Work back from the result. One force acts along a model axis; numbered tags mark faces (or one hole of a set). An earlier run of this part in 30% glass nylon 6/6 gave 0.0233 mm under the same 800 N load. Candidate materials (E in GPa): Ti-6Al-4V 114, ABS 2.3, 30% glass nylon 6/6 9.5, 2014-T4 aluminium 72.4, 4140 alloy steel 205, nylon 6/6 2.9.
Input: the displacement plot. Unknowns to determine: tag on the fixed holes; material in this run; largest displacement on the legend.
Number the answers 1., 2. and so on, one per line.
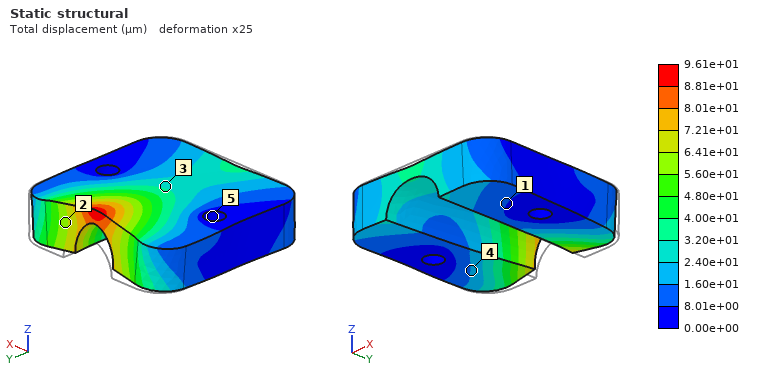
1. 5
2. ABS
3. 9.61e+01 µm
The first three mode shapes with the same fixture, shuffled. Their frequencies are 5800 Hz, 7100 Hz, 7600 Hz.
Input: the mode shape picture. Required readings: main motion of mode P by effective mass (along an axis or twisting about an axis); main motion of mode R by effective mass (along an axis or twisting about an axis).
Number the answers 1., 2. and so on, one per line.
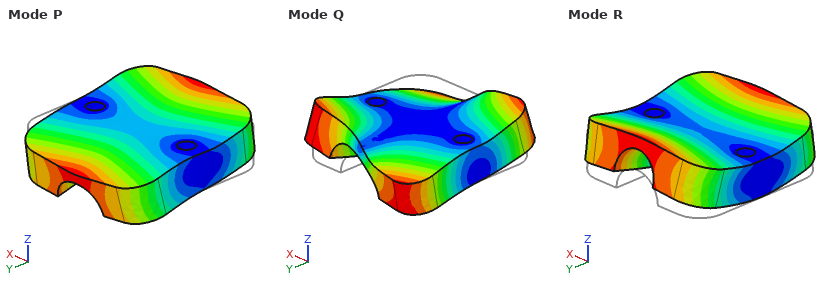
1. twisting about X
2. along Z
